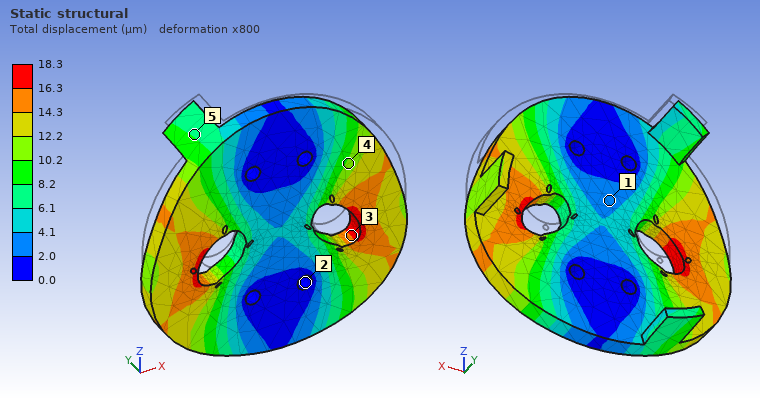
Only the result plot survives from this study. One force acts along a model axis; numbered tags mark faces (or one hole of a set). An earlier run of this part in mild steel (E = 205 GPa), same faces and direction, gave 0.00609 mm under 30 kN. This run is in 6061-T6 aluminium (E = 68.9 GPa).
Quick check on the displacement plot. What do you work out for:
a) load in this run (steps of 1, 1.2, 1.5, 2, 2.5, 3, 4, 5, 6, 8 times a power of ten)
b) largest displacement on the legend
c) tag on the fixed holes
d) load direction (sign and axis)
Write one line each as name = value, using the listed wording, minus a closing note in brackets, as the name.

load in this run = 30 kN
largest displacement on the legend = 18.3 µm
tag on the fixed holes = 2
load direction = -Z
